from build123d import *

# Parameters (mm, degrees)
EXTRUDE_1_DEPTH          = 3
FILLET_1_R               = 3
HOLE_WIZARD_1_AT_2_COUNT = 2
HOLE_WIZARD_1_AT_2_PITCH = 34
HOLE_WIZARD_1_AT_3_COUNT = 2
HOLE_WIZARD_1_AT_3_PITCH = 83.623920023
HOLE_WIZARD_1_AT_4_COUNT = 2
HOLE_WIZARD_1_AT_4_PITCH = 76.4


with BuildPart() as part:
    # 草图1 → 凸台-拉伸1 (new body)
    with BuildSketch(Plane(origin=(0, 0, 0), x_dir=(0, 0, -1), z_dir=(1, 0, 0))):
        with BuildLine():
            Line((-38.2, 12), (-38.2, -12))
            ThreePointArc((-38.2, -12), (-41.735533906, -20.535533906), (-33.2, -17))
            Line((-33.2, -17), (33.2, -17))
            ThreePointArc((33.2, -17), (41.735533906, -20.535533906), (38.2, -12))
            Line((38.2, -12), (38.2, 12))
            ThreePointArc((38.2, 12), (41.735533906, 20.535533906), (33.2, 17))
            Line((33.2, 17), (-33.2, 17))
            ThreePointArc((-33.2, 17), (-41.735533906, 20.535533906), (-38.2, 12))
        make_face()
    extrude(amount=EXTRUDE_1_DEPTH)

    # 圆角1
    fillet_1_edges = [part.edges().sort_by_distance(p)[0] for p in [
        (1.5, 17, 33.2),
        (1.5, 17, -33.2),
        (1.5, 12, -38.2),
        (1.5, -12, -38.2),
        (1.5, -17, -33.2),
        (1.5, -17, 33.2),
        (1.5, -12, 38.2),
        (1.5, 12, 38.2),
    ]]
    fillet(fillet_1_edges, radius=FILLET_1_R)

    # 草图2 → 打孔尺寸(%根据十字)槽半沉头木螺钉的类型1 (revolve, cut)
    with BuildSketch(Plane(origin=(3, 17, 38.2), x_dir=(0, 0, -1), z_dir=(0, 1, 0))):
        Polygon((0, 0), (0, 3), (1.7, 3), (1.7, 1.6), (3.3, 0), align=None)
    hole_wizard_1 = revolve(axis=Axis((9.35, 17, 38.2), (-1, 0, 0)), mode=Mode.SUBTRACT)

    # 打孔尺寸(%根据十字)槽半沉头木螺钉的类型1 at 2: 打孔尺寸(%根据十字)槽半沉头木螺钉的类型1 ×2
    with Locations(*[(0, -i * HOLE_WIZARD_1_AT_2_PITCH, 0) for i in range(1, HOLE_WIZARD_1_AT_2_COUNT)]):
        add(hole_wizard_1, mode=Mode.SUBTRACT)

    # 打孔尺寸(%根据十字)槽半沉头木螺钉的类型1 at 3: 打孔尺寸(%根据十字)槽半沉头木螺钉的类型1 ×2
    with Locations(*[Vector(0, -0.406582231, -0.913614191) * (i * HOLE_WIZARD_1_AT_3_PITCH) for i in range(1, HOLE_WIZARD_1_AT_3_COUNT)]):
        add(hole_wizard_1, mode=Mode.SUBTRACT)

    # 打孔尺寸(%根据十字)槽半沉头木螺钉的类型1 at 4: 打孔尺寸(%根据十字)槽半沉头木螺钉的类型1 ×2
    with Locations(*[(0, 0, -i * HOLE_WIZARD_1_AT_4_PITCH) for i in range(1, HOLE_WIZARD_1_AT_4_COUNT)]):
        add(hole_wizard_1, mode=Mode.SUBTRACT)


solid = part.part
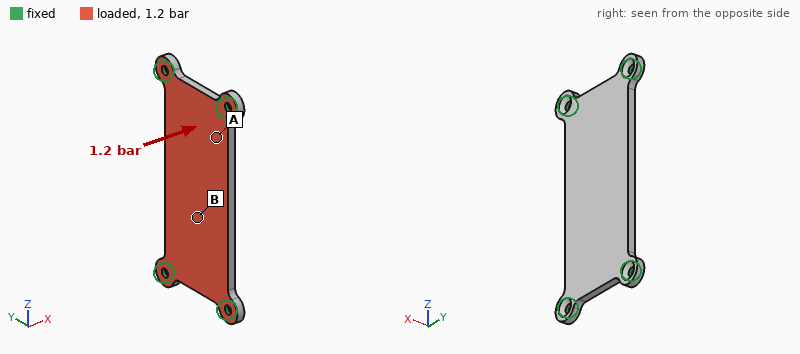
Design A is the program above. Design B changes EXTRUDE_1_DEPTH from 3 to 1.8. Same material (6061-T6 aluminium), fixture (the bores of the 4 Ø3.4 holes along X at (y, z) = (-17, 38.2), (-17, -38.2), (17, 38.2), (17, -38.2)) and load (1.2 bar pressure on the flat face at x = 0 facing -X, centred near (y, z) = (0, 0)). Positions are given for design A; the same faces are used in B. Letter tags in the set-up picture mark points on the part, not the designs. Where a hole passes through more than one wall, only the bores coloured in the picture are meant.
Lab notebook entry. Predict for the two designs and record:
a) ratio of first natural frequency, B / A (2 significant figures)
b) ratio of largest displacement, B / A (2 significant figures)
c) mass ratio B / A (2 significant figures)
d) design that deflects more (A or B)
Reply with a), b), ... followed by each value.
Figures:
a) 0.68
b) 3.6
c) 0.60
d) B
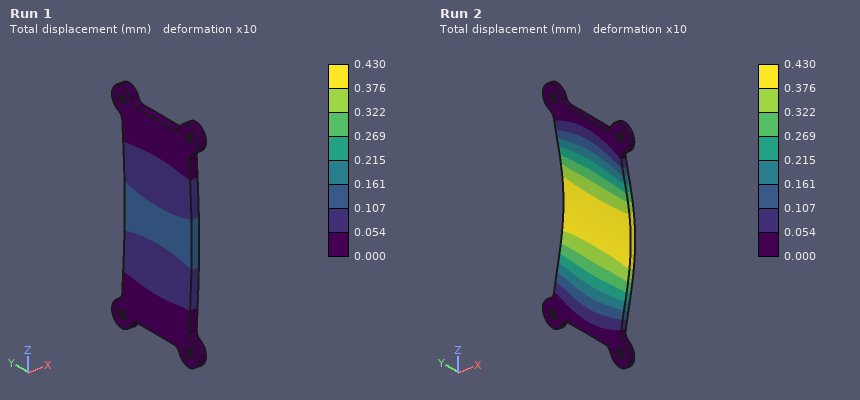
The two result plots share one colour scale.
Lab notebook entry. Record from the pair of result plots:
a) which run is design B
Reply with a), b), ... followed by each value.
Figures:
a) Run 2
